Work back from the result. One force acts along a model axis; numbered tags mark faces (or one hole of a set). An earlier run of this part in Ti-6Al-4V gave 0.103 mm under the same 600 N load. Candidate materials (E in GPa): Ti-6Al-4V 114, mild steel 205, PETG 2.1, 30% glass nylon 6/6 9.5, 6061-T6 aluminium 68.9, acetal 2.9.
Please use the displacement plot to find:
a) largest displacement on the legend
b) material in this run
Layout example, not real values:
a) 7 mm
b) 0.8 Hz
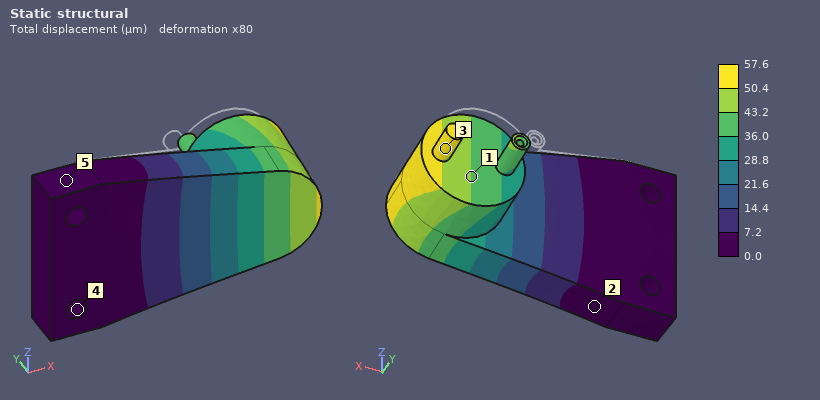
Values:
a) 57.6 µm
b) mild steel
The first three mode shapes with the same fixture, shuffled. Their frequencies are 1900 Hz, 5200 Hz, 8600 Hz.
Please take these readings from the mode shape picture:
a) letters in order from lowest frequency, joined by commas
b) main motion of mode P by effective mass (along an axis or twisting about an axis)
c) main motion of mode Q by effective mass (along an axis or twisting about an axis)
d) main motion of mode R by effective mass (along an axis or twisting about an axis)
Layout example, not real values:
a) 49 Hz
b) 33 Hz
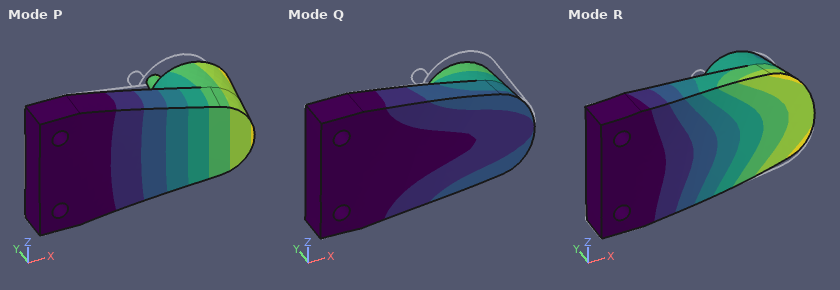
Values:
a) P, Q, R
b) along Y
c) along Z
d) along Z
